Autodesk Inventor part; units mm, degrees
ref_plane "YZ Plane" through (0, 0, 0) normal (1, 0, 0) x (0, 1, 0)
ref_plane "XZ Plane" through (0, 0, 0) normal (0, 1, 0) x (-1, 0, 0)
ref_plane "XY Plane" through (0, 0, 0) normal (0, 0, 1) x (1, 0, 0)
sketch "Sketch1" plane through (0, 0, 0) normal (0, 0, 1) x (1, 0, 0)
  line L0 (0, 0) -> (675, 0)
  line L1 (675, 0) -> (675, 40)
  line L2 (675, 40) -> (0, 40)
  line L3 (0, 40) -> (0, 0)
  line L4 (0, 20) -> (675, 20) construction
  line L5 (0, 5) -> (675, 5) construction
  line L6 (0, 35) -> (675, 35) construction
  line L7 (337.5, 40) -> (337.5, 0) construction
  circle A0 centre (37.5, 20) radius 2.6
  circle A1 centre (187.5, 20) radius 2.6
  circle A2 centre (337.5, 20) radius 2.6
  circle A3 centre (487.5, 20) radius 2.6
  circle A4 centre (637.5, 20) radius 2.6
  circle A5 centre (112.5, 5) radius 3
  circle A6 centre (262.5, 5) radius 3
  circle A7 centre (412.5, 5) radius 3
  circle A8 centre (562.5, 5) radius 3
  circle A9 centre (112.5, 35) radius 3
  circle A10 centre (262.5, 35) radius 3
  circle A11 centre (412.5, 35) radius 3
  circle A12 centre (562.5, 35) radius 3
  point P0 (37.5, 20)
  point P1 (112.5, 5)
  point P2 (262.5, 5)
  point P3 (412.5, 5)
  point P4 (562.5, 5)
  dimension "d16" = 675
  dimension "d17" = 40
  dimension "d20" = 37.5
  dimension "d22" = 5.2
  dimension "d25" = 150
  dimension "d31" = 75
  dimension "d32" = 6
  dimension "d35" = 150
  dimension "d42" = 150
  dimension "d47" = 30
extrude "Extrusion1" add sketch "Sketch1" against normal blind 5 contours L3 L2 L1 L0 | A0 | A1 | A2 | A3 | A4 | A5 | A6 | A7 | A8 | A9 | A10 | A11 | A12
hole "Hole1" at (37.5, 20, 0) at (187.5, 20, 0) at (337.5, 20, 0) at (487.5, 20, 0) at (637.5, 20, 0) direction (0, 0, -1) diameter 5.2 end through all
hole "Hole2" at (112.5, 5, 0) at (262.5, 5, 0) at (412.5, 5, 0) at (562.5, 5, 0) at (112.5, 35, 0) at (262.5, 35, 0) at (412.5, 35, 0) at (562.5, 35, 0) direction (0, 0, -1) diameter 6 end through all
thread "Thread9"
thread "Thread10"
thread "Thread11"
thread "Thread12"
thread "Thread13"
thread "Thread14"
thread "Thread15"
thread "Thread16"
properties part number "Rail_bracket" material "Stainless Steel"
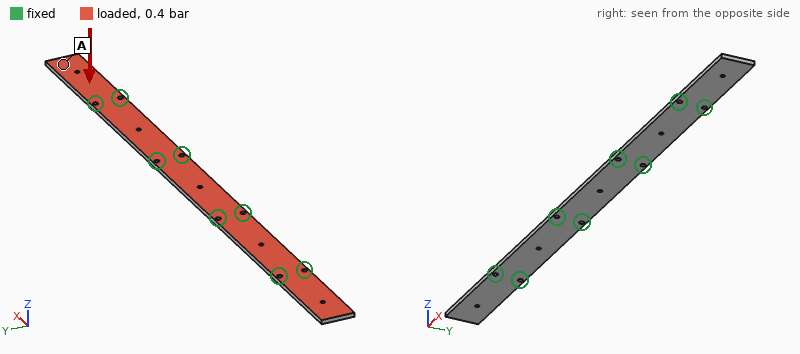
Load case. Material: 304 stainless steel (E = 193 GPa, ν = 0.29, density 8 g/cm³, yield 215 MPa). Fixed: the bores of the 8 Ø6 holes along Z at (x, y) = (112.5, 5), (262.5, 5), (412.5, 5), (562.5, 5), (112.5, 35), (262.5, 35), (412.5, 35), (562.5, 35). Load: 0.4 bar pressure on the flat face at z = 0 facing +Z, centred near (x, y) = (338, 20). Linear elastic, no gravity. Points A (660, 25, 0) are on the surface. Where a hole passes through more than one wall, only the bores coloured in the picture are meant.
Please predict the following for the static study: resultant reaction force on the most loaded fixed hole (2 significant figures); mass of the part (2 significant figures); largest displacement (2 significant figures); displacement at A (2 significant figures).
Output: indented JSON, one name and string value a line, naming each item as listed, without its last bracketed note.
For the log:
{
  "resultant reaction force on the most loaded fixed hole": "150 N",
  "mass of the part": "1.1 kg",
  "largest displacement": "0.38 mm",
  "displacement at A": "0.31 mm"
}
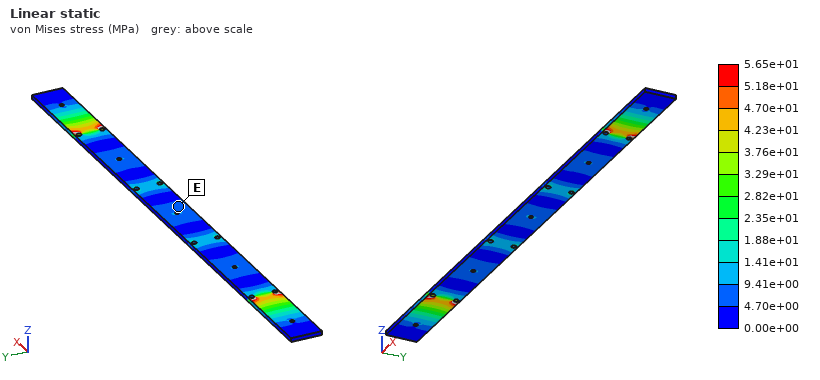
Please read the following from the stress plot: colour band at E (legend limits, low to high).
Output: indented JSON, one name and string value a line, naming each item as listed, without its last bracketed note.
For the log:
{
  "colour band at E": "4.70e+00 to 9.41e+00 MPa"
}
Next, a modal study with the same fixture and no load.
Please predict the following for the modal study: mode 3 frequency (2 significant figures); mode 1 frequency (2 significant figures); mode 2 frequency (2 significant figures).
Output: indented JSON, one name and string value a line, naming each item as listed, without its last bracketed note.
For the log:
{
  "mode 3 frequency": "1100 Hz",
  "mode 1 frequency": "320 Hz",
  "mode 2 frequency": "320 Hz"
}
